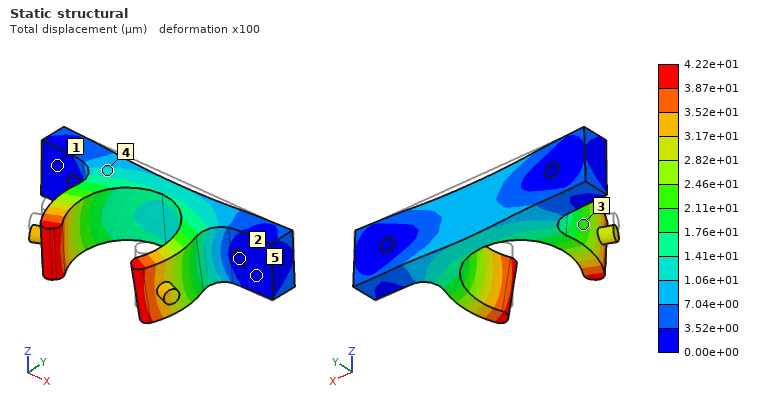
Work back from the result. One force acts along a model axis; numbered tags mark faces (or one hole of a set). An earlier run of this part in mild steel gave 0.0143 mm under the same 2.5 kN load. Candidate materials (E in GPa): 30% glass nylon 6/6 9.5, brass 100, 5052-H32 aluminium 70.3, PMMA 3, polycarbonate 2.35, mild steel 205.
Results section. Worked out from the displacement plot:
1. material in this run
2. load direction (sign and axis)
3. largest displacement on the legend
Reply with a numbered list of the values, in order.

1. 5052-H32 aluminium
2. -Z
3. 4.22e+01 µm
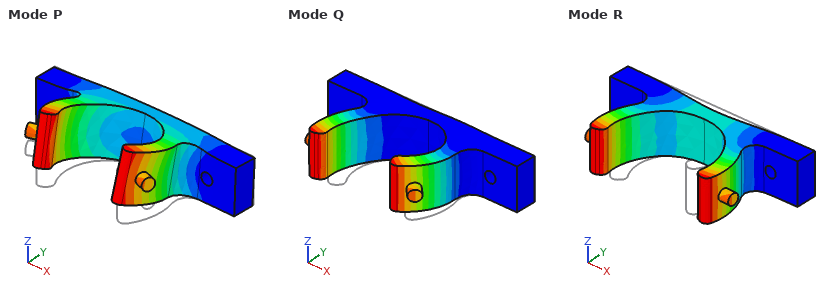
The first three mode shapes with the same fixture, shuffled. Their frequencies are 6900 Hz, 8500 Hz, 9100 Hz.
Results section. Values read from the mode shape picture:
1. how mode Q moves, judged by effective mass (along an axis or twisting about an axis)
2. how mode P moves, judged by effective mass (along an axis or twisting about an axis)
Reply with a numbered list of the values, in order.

1. along X
2. along Z
